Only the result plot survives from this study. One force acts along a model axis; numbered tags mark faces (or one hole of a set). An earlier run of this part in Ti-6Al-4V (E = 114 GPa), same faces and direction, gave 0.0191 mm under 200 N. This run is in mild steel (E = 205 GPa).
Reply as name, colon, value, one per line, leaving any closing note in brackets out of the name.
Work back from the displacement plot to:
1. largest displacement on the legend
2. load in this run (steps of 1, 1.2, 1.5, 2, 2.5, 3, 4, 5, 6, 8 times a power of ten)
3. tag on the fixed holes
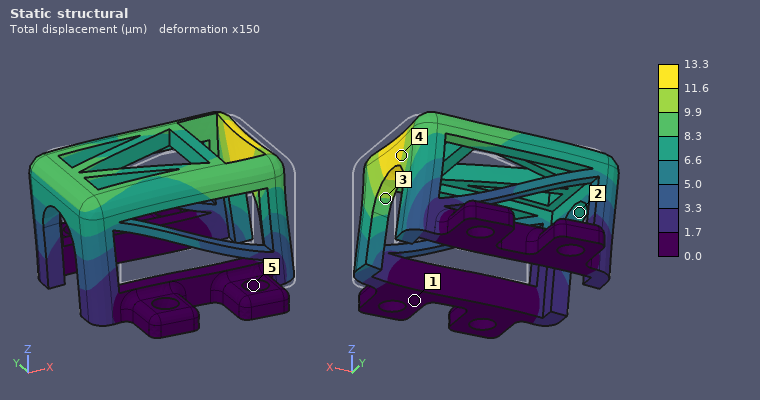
largest displacement on the legend: 13.3 µm
load in this run: 250 N
tag on the fixed holes: 5
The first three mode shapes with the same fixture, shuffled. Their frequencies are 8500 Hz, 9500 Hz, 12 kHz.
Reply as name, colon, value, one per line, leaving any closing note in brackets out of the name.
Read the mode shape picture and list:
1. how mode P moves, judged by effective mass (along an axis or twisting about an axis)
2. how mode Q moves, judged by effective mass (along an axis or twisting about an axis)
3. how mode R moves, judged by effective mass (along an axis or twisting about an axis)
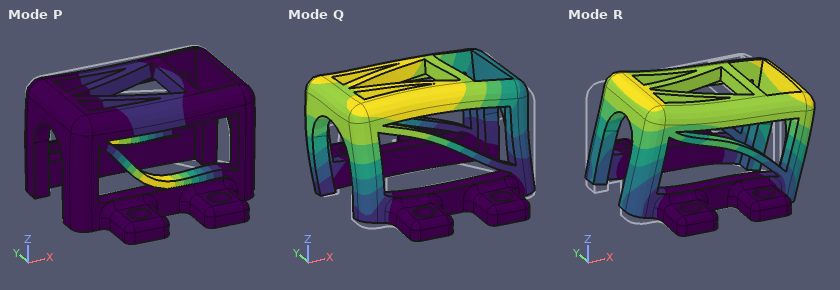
how mode P moves, judged by effective mass: along Z
how mode Q moves, judged by effective mass: along Y
how mode R moves, judged by effective mass: along X
